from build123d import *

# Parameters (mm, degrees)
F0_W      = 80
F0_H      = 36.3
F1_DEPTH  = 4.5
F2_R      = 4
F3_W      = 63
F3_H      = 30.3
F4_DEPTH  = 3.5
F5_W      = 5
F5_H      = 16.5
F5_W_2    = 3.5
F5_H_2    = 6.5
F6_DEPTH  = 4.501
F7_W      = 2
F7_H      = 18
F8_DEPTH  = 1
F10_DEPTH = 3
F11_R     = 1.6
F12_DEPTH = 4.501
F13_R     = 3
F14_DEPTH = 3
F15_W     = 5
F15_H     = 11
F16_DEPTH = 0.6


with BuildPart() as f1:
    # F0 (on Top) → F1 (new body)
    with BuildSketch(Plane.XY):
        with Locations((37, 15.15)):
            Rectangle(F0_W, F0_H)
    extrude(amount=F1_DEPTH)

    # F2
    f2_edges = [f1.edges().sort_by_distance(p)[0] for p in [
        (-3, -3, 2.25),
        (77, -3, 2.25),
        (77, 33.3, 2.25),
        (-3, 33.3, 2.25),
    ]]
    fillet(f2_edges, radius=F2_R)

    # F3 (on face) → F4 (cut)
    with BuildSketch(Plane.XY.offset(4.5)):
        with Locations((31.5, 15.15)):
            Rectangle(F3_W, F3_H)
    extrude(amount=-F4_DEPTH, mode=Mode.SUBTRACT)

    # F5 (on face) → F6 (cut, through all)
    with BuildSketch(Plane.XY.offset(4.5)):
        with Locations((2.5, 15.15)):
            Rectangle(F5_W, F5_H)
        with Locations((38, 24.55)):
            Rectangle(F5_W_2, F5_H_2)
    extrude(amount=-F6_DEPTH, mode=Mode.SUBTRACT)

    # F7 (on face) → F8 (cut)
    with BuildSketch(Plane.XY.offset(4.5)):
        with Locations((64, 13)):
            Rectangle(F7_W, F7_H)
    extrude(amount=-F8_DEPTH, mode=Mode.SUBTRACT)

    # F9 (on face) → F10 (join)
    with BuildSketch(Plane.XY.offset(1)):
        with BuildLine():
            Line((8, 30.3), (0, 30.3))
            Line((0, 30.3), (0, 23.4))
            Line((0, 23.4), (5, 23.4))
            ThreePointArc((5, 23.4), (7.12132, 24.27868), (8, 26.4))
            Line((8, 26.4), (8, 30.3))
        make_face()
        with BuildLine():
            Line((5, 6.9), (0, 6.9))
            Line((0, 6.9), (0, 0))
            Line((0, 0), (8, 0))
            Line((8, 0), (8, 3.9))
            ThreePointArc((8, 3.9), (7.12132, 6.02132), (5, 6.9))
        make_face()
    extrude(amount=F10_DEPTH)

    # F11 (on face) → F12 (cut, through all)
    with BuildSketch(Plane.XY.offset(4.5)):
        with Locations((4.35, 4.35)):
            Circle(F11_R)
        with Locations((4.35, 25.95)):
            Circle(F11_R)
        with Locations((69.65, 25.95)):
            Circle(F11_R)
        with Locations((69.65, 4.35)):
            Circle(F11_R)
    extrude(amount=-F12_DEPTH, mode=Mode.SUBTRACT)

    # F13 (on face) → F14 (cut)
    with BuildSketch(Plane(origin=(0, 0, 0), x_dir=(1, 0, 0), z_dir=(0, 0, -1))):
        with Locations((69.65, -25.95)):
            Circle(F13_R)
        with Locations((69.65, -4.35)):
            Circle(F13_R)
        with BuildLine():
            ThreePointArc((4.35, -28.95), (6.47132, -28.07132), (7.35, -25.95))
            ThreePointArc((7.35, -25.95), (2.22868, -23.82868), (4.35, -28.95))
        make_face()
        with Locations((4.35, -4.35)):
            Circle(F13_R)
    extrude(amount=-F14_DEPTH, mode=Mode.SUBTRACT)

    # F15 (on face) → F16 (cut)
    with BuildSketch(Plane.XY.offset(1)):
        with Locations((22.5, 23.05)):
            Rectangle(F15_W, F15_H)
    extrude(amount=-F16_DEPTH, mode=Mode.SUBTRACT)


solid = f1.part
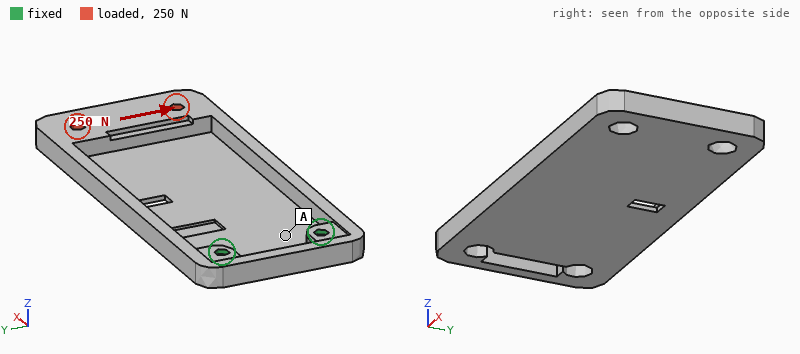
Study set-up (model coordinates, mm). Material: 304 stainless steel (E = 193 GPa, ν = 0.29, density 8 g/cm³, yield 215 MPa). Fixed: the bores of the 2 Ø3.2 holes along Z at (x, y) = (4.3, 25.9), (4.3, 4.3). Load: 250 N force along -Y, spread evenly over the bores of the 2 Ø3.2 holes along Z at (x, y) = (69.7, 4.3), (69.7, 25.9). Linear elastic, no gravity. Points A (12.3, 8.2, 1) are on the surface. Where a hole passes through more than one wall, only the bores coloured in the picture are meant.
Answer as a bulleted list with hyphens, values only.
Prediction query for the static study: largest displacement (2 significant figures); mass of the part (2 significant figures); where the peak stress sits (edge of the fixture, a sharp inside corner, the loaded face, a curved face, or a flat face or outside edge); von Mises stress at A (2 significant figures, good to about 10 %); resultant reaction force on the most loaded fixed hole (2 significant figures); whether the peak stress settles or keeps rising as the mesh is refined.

- 0.17 mm
- 49 g
- edge of the fixture
- 30 MPa
- 550 N
- keeps rising
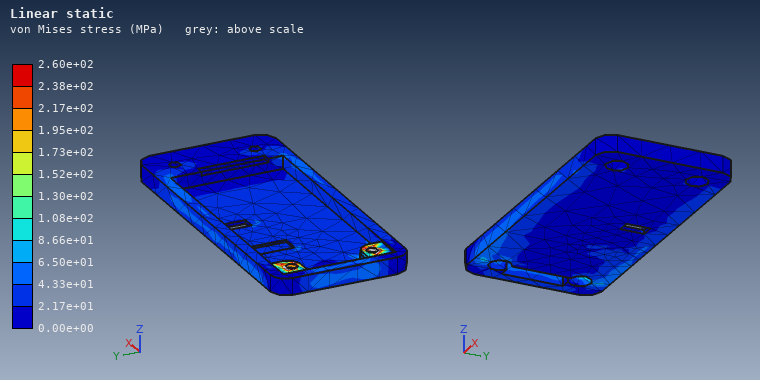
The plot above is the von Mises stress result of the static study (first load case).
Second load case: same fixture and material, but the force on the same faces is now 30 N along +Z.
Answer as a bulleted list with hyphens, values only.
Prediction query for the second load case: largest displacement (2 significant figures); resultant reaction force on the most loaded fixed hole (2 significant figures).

- 0.37 mm
- 69 N
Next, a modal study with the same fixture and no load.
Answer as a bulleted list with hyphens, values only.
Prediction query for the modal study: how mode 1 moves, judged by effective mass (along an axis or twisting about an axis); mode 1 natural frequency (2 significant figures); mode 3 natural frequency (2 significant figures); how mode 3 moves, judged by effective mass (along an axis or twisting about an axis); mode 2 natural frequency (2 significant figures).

- along Z
- 330 Hz
- 2400 Hz
- along Y
- 1100 Hz
